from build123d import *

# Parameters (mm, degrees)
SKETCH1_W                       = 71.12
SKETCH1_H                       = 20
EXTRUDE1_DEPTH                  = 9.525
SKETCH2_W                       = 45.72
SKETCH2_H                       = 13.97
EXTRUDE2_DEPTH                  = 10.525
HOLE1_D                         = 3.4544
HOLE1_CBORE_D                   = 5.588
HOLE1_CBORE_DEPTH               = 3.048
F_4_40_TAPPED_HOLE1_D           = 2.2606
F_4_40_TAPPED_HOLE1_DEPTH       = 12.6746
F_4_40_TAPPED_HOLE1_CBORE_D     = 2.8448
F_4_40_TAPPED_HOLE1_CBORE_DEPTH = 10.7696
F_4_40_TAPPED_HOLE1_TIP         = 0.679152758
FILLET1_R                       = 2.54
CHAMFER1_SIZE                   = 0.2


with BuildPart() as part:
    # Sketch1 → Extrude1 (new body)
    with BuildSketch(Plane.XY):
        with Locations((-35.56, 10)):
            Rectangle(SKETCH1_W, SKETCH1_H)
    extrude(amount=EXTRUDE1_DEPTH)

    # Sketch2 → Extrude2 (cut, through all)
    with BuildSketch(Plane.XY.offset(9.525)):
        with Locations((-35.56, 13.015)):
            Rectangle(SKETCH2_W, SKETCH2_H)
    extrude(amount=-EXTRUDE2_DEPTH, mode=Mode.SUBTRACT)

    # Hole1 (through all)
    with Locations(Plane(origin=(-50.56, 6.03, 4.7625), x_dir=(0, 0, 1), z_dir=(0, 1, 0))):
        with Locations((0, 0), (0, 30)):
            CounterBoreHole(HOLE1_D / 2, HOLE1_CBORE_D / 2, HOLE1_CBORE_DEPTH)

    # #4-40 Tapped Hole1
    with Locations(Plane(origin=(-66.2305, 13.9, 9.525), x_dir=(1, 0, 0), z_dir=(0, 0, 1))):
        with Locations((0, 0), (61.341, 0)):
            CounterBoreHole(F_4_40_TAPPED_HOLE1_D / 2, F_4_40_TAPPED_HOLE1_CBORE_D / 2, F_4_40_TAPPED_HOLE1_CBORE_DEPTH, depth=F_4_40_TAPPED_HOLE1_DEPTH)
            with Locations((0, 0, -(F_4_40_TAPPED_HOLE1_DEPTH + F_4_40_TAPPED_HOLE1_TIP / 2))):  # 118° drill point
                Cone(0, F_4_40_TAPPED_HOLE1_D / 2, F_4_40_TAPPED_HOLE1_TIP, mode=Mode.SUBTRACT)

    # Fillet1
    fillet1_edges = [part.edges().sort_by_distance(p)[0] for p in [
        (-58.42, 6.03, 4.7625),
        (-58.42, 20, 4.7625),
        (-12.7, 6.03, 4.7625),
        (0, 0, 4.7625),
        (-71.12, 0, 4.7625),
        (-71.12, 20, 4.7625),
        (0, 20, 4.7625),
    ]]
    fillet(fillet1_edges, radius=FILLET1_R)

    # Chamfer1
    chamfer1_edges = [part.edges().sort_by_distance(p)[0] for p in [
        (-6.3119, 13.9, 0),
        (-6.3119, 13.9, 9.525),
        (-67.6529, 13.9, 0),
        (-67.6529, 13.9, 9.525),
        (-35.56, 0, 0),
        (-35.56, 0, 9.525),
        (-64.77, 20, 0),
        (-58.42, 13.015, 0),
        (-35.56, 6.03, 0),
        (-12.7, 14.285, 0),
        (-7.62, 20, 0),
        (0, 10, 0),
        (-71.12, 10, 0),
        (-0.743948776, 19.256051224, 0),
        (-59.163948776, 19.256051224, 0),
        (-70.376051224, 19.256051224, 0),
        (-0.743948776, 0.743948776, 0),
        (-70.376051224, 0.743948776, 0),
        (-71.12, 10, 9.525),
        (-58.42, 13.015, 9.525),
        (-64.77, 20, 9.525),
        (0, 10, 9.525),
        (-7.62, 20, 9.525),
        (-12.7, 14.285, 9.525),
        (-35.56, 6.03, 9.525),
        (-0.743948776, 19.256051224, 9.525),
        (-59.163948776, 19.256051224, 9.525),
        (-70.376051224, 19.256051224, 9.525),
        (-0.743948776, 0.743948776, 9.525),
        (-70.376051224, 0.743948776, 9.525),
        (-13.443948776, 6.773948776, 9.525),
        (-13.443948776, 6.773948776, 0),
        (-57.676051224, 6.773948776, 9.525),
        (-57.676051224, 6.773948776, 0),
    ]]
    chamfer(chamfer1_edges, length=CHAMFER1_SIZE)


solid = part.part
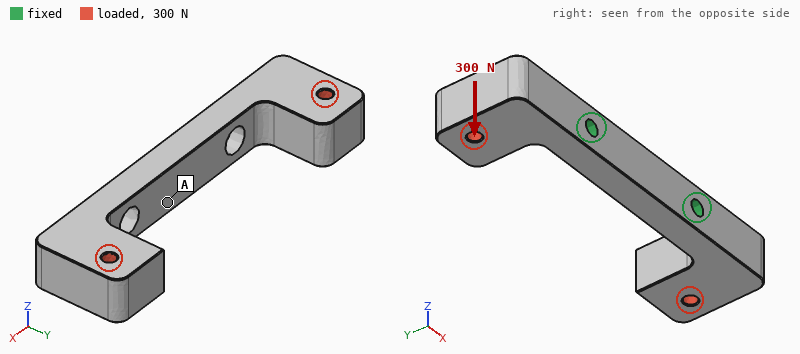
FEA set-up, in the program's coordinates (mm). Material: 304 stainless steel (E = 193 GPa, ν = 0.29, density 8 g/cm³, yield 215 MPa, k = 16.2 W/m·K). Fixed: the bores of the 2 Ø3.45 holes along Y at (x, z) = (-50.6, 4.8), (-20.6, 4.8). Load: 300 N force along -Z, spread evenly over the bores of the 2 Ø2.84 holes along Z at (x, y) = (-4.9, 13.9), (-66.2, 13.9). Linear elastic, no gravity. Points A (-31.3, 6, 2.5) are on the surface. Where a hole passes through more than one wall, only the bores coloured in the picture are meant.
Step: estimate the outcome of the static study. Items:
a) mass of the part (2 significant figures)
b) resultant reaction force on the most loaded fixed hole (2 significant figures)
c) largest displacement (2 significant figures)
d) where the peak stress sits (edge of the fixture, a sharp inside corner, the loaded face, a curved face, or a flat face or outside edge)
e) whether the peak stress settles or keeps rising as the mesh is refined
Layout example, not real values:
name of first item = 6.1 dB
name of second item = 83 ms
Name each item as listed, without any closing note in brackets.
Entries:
mass of the part = 57 g
resultant reaction force on the most loaded fixed hole = 150 N
largest displacement = 18 µm
where the peak stress sits = edge of the fixture
whether the peak stress settles or keeps rising as the mesh is refined = keeps rising
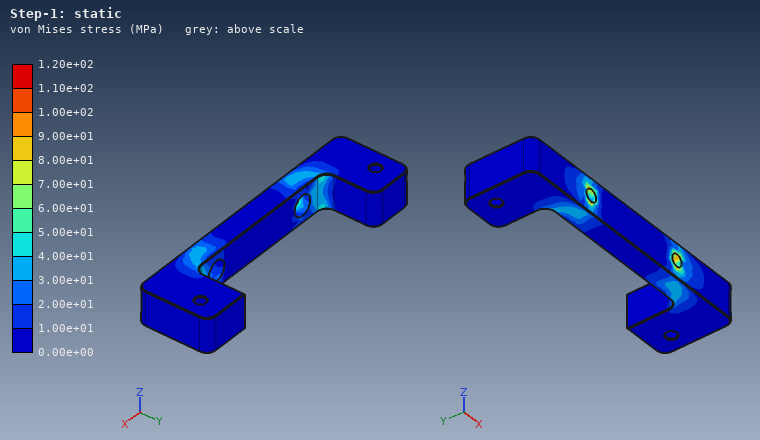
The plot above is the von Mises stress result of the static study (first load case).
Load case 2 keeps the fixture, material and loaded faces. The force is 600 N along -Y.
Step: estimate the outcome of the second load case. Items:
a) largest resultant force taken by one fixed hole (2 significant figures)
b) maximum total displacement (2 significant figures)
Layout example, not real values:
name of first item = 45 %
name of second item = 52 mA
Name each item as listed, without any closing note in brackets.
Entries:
largest resultant force taken by one fixed hole = 520 N
maximum total displacement = 37 µm
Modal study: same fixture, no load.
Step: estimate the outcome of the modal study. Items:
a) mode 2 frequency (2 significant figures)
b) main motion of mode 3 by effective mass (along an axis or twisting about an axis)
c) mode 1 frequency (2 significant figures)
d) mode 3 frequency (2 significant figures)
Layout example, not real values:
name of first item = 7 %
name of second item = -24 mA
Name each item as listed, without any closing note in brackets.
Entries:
mode 2 frequency = 3800 Hz
main motion of mode 3 by effective mass = along Z
mode 1 frequency = 3800 Hz
mode 3 frequency = 4800 Hz
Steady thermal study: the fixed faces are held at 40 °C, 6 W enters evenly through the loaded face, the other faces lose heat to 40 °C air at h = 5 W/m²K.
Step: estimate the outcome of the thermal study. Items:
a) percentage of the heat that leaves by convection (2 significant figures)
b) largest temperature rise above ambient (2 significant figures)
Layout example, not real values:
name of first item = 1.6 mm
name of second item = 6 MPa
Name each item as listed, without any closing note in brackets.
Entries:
percentage of the heat that leaves by convection = 8.2 %
largest temperature rise above ambient = 54 K
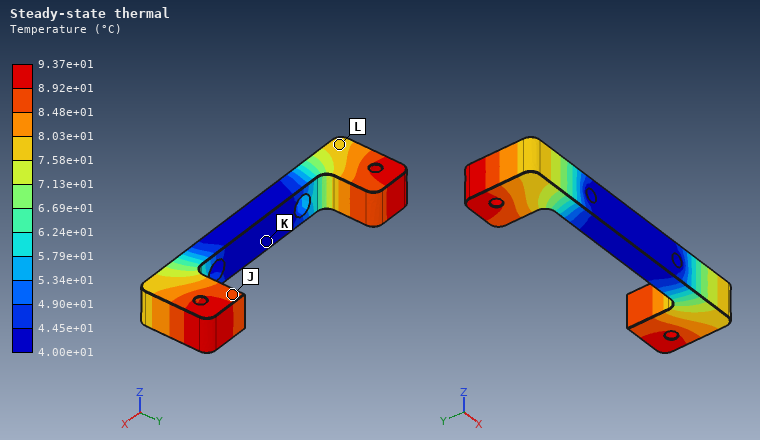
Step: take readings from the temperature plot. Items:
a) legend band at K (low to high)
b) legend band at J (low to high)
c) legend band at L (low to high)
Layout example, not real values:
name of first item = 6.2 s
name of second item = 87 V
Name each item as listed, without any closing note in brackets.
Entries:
legend band at K = 4.00e+01 to 4.45e+01 °C
legend band at J = 8.48e+01 to 8.92e+01 °C
legend band at L = 7.58e+01 to 8.03e+01 °C
